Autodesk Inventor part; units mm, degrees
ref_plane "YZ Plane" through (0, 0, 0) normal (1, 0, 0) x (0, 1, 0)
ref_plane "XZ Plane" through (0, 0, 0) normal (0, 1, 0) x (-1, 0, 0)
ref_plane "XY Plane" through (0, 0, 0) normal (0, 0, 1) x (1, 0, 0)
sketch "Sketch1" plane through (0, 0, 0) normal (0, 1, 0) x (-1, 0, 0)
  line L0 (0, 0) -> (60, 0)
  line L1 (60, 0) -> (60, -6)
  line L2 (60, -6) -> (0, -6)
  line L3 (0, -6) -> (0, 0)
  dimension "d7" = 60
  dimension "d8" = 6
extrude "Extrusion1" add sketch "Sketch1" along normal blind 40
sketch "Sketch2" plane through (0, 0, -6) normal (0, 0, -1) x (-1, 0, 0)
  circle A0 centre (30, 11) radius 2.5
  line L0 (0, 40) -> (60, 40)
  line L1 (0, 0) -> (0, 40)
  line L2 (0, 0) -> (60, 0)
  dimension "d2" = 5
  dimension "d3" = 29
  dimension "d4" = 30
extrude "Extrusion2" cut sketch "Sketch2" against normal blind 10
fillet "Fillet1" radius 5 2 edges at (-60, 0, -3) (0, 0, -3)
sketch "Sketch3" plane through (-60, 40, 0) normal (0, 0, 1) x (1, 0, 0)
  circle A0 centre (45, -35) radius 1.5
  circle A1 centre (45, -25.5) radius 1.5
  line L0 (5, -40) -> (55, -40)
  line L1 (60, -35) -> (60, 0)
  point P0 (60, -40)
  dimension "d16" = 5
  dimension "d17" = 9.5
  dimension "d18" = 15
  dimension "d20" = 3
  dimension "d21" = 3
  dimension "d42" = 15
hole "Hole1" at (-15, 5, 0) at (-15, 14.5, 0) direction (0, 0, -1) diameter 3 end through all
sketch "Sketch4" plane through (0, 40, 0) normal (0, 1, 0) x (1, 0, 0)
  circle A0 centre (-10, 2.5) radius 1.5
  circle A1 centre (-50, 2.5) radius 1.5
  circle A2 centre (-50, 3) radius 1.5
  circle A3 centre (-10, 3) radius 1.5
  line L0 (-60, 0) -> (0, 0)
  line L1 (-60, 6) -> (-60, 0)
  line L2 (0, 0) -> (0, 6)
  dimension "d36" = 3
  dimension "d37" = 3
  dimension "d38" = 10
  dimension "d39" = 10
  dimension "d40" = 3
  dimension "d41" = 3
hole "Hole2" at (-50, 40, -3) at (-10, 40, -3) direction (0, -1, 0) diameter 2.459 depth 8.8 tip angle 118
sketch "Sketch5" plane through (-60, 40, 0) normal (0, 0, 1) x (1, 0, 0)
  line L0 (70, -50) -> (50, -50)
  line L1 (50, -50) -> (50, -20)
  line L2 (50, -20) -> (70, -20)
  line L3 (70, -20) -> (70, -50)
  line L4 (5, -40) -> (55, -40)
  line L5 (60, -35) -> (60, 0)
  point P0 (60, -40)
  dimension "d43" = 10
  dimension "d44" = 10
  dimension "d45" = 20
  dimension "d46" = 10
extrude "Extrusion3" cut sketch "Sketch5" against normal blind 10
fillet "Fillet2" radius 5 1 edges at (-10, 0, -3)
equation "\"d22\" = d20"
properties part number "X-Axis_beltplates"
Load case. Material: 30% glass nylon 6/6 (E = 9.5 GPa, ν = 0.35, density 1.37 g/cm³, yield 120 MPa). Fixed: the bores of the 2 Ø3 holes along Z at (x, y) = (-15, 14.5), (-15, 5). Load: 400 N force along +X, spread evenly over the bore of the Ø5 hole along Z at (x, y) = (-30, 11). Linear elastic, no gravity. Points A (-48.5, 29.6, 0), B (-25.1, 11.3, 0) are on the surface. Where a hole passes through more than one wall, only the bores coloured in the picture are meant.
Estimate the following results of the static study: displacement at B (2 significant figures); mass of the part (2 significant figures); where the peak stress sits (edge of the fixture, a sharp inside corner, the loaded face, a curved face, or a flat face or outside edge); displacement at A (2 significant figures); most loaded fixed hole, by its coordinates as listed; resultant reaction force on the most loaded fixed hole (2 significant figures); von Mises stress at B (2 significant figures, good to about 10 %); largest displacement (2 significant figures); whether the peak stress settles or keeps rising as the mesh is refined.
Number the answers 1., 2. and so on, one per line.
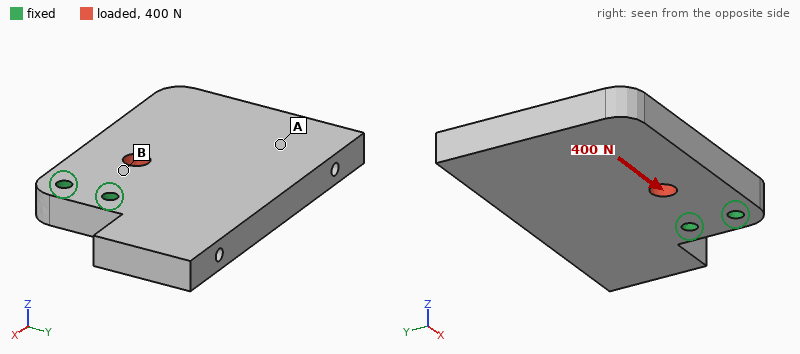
1. 4.3 µm
2. 18 g
3. edge of the fixture
4. 6.5 µm
5. (-15, 14.5)
6. 250 N
7. 4.6 MPa
8. 8.3 µm
9. keeps rising
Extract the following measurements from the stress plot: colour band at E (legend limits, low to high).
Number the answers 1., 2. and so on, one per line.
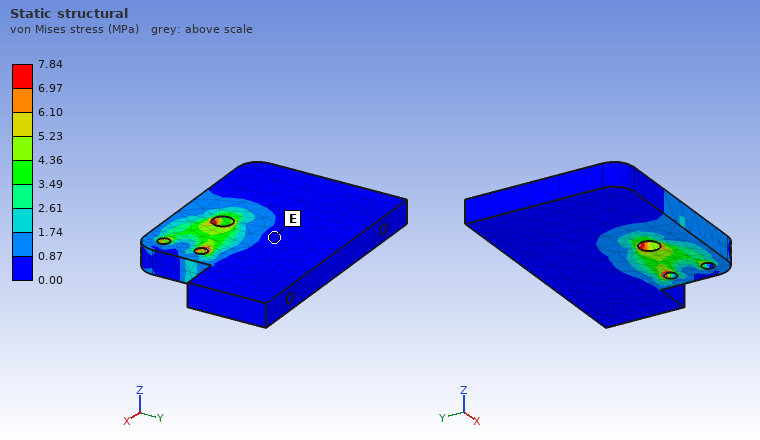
1. 0.00 to 0.87 MPa
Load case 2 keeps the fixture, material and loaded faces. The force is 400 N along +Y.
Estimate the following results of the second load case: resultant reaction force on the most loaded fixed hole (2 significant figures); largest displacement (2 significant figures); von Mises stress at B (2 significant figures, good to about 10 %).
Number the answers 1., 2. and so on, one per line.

1. 530 N
2. 97 µm
3. 9.9 MPa
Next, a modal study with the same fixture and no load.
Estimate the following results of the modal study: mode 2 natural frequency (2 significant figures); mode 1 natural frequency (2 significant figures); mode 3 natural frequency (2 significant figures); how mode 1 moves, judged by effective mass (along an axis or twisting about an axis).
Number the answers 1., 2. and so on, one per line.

1. 2200 Hz
2. 1000 Hz
3. 2300 Hz
4. along Z
